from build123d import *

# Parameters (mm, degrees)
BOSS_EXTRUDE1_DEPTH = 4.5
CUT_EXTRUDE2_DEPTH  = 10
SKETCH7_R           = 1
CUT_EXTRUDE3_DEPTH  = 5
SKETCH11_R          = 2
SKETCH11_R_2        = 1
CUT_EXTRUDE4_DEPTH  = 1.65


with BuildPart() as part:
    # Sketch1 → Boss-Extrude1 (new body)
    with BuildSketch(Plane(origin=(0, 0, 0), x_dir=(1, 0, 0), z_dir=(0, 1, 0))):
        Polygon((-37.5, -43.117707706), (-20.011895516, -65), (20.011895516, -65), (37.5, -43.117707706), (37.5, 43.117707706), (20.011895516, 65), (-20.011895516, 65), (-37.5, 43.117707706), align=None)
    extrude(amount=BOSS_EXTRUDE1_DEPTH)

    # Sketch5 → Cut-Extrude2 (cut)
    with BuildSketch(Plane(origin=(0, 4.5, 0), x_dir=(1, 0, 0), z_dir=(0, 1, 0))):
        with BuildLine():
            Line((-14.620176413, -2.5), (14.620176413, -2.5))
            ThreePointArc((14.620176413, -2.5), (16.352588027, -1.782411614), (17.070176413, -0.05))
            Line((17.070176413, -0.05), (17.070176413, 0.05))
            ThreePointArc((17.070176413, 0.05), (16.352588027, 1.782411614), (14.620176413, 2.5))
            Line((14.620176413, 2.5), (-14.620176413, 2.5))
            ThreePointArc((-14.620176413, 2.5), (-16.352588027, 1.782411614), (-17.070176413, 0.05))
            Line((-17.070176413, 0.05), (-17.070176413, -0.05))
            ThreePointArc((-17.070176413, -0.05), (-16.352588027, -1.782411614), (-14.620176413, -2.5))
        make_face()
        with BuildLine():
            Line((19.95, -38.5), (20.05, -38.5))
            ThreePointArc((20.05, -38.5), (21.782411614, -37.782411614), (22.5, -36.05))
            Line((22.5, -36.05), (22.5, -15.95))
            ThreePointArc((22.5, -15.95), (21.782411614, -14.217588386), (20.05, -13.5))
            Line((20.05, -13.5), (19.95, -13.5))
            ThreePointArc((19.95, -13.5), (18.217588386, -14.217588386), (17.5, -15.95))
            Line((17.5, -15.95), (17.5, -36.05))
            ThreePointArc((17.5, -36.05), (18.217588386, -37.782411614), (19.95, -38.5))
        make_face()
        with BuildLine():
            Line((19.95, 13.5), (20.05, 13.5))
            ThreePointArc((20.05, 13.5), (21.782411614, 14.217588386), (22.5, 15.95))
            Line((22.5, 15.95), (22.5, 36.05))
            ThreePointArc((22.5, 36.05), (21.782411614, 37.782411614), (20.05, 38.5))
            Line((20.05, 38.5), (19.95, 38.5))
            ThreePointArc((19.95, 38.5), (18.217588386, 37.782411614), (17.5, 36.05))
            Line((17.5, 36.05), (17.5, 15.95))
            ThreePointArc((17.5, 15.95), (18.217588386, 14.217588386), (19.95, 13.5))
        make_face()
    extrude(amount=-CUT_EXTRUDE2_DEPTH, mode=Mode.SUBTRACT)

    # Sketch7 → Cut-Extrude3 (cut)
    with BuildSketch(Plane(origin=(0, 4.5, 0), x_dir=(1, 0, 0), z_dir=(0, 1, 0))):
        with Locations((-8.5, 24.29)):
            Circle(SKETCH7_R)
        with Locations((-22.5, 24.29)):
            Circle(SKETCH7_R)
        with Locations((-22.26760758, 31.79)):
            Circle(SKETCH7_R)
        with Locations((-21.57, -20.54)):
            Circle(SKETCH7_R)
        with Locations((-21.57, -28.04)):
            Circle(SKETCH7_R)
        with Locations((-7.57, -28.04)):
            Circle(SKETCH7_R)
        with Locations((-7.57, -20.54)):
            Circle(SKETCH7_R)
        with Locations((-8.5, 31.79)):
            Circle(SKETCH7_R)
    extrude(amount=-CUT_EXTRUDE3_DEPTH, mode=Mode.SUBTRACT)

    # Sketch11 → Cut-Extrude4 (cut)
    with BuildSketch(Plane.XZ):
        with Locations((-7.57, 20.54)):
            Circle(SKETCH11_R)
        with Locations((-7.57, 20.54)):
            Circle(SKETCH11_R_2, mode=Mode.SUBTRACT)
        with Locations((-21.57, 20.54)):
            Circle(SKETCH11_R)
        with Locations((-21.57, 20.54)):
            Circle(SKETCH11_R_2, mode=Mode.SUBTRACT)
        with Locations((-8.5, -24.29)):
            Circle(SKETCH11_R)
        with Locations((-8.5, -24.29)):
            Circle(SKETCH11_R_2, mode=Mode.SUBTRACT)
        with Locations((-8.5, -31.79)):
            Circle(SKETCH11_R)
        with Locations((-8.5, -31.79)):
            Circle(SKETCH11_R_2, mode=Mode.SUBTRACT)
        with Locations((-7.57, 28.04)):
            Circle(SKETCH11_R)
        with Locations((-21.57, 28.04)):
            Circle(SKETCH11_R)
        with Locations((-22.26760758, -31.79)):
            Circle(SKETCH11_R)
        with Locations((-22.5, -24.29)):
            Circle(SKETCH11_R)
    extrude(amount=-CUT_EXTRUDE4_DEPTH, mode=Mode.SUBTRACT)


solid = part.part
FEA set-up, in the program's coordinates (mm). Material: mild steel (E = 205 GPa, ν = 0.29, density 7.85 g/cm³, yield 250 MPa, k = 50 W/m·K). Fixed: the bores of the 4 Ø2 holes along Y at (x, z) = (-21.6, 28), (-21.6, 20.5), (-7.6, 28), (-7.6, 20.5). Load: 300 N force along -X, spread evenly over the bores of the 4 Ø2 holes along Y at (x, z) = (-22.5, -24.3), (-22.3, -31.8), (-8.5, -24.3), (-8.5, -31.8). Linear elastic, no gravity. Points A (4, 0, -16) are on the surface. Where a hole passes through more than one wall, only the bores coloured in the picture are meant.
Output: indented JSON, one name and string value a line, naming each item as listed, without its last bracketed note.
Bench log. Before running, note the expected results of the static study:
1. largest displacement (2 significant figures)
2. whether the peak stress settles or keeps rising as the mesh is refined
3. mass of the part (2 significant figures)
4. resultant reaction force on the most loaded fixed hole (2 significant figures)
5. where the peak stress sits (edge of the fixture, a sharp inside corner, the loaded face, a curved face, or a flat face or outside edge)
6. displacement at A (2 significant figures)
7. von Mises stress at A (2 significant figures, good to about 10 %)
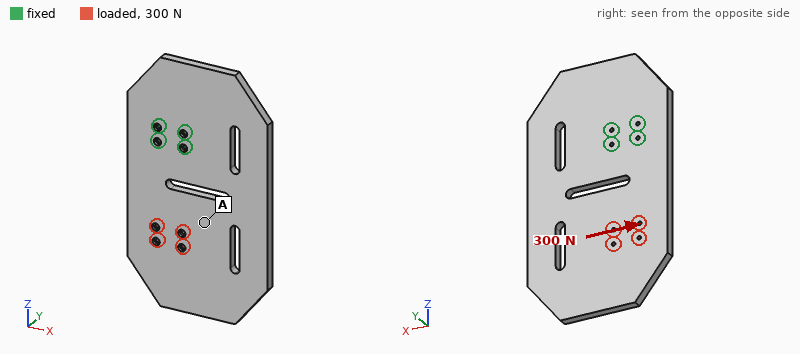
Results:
{
  "largest displacement": "10 µm",
  "whether the peak stress settles or keeps rising as the mesh is refined": "keeps rising",
  "mass of the part": "300 g",
  "resultant reaction force on the most loaded fixed hole": "550 N",
  "where the peak stress sits": "edge of the fixture",
  "displacement at A": "4.7 µm",
  "von Mises stress at A": "1.8 MPa"
}
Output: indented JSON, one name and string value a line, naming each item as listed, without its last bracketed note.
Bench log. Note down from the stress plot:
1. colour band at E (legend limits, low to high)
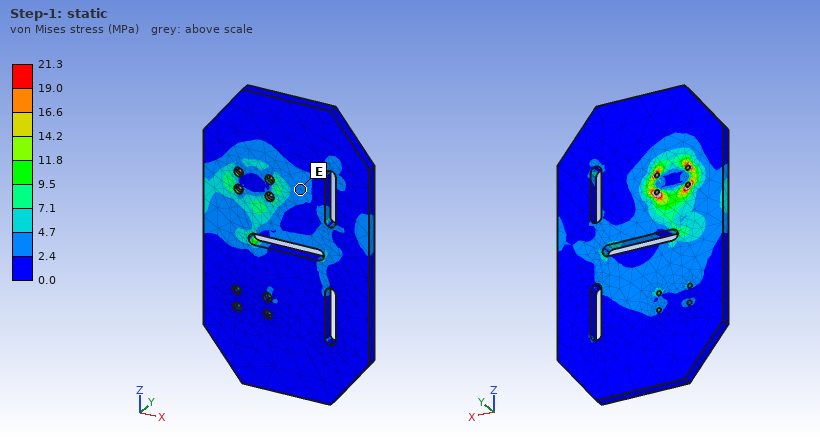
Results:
{
  "colour band at E": "2.4 to 4.7 MPa"
}
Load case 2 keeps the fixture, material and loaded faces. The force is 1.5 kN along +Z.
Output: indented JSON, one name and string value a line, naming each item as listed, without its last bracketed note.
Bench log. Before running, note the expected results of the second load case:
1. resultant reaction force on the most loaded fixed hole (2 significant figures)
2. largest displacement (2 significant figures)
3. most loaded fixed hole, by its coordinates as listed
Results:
{
  "resultant reaction force on the most loaded fixed hole": "560 N",
  "largest displacement": "49 µm",
  "most loaded fixed hole, by its coordinates as listed": "(-21.6, 20.5)"
}
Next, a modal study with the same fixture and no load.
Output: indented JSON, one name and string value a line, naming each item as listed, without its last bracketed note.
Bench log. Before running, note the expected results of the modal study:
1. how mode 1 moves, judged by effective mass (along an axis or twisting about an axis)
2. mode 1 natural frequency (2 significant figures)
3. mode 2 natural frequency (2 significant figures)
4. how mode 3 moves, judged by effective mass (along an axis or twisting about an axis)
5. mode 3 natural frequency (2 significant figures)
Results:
{
  "how mode 1 moves, judged by effective mass": "along Y",
  "mode 1 natural frequency": "410 Hz",
  "mode 2 natural frequency": "1100 Hz",
  "how mode 3 moves, judged by effective mass": "along Y",
  "mode 3 natural frequency": "1700 Hz"
}
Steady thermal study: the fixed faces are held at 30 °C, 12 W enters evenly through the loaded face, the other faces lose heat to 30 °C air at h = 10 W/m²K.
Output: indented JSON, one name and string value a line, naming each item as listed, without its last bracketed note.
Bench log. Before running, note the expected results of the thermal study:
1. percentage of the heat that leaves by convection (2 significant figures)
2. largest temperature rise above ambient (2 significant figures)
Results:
{
  "percentage of the heat that leaves by convection": "37 %",
  "largest temperature rise above ambient": "54 K"
}
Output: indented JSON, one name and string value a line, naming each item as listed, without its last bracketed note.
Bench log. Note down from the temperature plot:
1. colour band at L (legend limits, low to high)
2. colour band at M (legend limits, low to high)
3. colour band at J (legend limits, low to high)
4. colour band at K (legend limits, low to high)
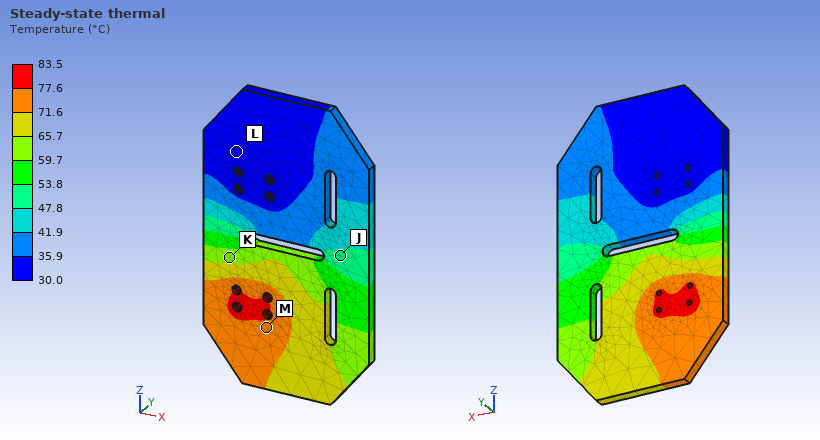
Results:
{
  "colour band at L": "30.0 to 35.9 °C",
  "colour band at M": "71.6 to 77.6 °C",
  "colour band at J": "47.8 to 53.8 °C",
  "colour band at K": "59.7 to 65.7 °C"
}
